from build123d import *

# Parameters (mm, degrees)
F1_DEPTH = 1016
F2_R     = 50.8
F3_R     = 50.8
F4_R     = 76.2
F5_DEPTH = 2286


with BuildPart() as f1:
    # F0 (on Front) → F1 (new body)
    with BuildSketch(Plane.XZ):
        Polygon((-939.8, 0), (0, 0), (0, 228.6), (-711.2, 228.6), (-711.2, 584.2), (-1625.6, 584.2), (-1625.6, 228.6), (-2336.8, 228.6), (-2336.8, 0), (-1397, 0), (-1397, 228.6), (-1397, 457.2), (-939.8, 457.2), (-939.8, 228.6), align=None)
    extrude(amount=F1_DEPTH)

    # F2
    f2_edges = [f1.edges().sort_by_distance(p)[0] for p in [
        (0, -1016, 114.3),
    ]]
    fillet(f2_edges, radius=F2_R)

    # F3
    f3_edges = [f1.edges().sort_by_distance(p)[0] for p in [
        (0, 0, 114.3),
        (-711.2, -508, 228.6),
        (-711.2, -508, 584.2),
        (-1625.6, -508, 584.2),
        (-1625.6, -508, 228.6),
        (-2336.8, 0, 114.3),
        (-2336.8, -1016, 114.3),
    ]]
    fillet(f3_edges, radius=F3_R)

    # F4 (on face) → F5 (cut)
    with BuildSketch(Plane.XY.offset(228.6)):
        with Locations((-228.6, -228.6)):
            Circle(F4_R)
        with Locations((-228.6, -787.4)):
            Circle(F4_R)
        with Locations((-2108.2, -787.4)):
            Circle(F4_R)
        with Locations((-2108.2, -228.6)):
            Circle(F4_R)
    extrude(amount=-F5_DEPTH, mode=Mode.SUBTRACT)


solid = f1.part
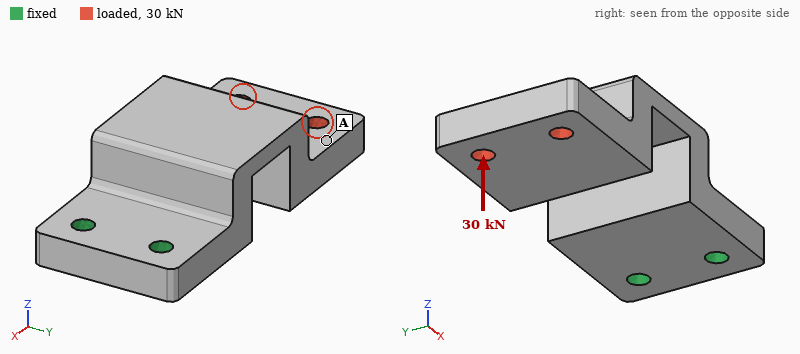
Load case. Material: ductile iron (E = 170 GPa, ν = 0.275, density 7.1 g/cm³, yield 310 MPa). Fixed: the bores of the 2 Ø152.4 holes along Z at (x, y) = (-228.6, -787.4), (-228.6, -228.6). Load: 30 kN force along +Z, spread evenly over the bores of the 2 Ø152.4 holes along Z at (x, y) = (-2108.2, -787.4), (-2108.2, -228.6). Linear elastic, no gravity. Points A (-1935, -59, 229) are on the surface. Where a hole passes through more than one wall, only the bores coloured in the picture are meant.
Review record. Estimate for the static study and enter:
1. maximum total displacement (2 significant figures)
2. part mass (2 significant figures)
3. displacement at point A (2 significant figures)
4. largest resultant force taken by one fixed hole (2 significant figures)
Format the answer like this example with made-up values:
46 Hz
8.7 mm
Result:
1.1 mm
4600 kg
0.74 mm
15 kN
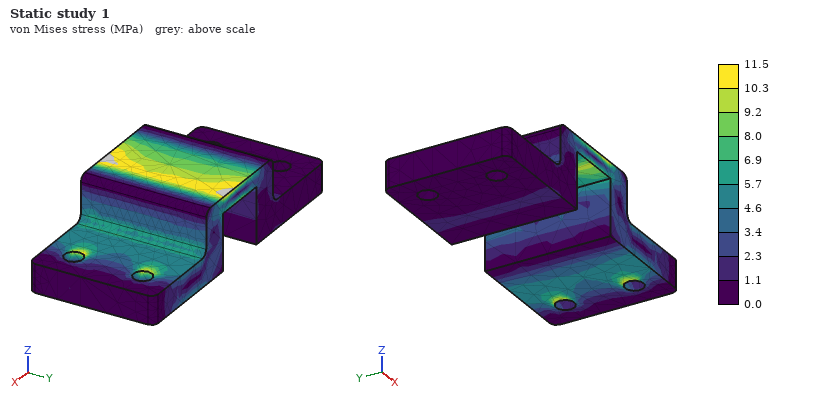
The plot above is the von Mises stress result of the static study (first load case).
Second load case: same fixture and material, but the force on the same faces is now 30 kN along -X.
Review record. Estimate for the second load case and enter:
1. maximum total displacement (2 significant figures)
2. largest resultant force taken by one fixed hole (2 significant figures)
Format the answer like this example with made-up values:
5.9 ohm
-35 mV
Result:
0.32 mm
15 kN
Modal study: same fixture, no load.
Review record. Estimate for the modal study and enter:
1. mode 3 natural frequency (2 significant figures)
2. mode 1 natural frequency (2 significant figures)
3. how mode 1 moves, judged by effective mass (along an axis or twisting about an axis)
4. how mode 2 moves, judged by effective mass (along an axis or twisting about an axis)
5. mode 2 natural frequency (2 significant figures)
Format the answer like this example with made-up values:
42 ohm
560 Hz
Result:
87 Hz
26 Hz
along Z
along Y
64 Hz
